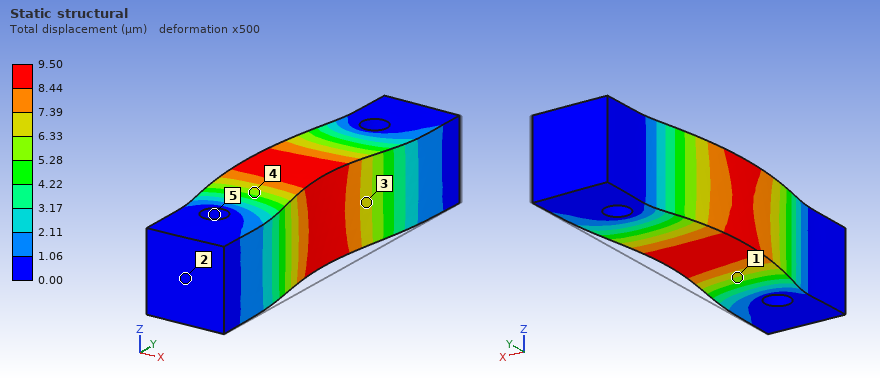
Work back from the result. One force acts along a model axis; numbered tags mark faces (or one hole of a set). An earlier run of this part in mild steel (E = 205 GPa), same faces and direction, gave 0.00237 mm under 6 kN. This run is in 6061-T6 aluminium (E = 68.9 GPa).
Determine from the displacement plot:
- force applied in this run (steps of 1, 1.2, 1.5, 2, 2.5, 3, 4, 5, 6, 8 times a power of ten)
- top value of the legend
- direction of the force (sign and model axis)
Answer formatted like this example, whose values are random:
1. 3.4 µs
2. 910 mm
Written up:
1. 8 kN
2. 9.50 µm
3. -X
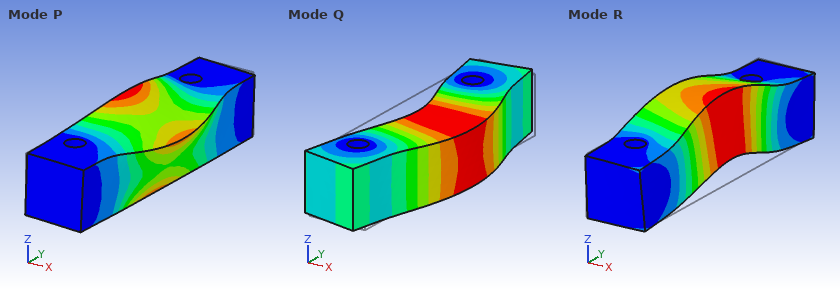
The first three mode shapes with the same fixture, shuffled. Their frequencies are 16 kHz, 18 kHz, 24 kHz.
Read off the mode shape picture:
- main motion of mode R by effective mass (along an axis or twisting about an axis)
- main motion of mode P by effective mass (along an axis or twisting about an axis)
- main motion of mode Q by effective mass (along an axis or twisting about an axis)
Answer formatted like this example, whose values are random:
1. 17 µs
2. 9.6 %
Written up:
1. along Z
2. twisting about Y
3. along X
